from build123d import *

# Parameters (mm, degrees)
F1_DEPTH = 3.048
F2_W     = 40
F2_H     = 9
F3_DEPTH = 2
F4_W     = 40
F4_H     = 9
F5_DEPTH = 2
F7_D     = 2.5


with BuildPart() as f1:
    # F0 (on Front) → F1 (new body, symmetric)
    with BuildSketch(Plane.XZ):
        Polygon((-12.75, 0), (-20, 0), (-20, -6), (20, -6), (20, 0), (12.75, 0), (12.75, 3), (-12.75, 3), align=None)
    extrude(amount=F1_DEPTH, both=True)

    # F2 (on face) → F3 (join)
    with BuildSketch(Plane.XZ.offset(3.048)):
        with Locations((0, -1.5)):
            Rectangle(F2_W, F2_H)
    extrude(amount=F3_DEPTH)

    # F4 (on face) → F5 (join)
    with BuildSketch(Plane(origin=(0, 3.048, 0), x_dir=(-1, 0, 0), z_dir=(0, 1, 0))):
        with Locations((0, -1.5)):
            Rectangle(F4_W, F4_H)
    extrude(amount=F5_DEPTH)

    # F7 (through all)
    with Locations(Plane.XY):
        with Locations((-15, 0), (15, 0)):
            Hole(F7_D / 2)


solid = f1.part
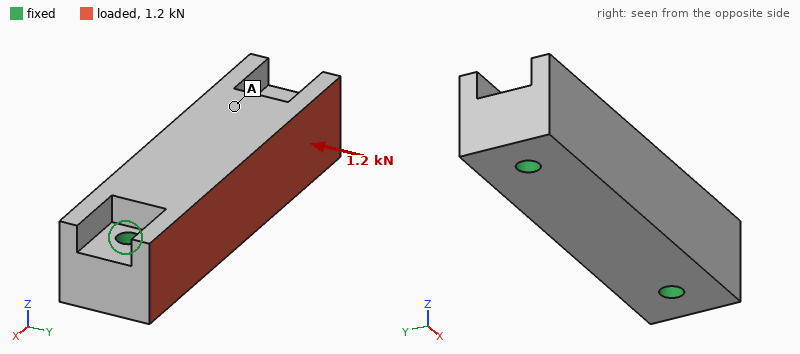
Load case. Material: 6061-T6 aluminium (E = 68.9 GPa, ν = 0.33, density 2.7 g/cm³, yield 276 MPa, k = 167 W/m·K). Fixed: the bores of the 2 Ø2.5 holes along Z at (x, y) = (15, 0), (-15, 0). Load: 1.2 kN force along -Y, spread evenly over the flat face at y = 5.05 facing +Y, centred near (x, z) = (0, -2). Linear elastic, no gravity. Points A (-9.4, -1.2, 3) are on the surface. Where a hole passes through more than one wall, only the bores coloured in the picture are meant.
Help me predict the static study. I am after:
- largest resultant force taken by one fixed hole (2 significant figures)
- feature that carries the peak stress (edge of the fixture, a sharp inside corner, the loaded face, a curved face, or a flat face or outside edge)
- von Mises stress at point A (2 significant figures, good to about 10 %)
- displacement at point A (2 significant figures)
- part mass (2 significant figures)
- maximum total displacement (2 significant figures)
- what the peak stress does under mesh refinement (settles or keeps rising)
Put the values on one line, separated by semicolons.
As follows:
600 N; edge of the fixture; 8.2 MPa; 4.0 µm; 8.9 g; 6.4 µm; keeps rising
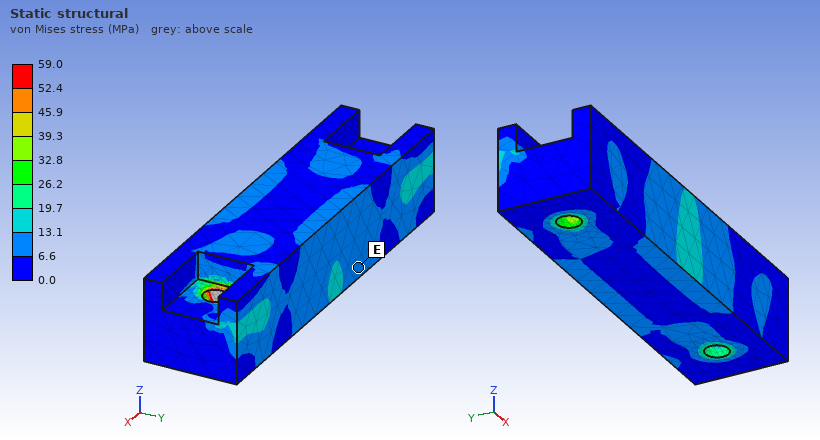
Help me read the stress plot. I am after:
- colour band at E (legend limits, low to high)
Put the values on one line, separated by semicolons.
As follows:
6.6 to 13.1 MPa
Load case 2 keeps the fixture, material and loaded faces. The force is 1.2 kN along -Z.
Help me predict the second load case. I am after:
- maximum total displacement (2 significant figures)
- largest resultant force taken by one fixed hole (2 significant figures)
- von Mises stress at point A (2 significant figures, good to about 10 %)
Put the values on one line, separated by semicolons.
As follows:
12 µm; 620 N; 14 MPa
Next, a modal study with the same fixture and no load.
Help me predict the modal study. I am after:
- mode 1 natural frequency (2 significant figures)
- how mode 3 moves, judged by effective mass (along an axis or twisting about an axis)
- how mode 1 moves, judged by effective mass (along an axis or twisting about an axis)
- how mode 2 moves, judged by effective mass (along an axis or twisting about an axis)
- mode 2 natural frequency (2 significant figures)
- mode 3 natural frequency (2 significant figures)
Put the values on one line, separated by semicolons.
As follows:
26 kHz; twisting about X; along Y; along Z; 28 kHz; 36 kHz
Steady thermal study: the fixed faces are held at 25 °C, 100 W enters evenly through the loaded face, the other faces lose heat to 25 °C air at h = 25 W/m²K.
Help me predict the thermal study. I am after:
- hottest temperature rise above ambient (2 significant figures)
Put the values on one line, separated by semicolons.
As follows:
30 K
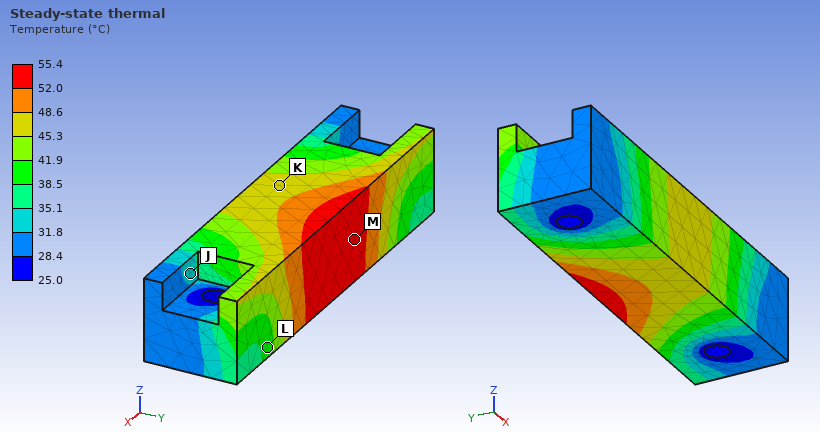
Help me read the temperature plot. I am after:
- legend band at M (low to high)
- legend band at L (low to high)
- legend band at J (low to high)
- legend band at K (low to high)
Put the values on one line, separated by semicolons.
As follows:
52.0 to 55.4 °C; 38.5 to 41.9 °C; 31.8 to 35.1 °C; 45.3 to 48.6 °C
